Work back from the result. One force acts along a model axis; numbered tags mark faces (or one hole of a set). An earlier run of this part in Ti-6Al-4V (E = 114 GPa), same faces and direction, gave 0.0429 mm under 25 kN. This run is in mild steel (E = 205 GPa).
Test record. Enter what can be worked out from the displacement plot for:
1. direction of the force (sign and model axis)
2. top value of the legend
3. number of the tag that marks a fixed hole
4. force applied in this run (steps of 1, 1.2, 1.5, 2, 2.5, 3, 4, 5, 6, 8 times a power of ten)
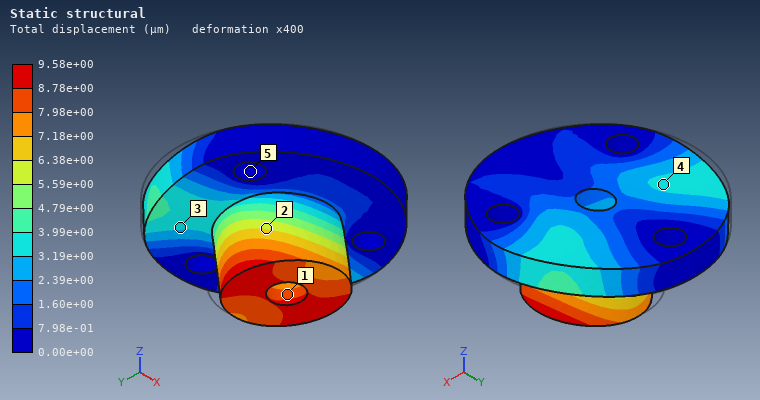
+X
9.58e+00 µm
5
10 kN
